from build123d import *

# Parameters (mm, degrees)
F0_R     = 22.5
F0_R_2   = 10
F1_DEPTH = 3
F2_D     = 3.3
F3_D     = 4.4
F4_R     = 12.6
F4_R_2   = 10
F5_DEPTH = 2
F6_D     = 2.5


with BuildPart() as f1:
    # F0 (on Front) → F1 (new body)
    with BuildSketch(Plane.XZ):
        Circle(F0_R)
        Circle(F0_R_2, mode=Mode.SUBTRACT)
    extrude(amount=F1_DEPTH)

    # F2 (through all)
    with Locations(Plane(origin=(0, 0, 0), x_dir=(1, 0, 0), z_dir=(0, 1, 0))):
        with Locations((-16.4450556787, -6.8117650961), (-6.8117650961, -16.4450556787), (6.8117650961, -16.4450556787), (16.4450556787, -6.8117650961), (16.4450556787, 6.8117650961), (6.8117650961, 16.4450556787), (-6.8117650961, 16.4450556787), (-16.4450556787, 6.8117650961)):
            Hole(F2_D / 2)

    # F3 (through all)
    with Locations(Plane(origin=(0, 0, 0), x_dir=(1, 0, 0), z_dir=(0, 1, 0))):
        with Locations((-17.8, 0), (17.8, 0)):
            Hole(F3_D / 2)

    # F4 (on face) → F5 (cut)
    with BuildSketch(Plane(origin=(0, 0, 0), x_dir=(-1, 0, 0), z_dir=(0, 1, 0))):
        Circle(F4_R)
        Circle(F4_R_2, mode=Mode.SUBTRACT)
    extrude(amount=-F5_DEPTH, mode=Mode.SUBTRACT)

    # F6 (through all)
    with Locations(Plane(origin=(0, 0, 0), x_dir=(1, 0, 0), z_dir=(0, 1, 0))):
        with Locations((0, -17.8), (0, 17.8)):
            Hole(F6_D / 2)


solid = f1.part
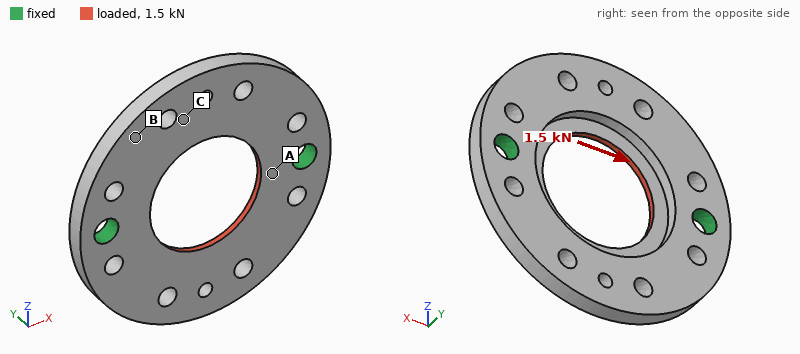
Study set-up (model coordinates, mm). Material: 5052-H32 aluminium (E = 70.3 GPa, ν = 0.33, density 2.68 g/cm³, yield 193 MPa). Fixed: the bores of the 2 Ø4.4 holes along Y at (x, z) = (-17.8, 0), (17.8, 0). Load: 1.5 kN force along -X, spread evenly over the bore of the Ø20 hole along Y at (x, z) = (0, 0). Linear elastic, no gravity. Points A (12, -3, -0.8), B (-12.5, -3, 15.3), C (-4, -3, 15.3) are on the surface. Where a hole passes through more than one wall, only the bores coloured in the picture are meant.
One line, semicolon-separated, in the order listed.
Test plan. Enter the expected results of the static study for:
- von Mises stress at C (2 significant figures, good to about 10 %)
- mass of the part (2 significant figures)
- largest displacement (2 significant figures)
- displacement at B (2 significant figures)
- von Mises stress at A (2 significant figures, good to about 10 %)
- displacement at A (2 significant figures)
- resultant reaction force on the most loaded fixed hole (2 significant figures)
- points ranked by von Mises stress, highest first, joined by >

12 MPa; 8.4 g; 10 µm; 7.9 µm; 40 MPa; 2.8 µm; 750 N; A > C > B
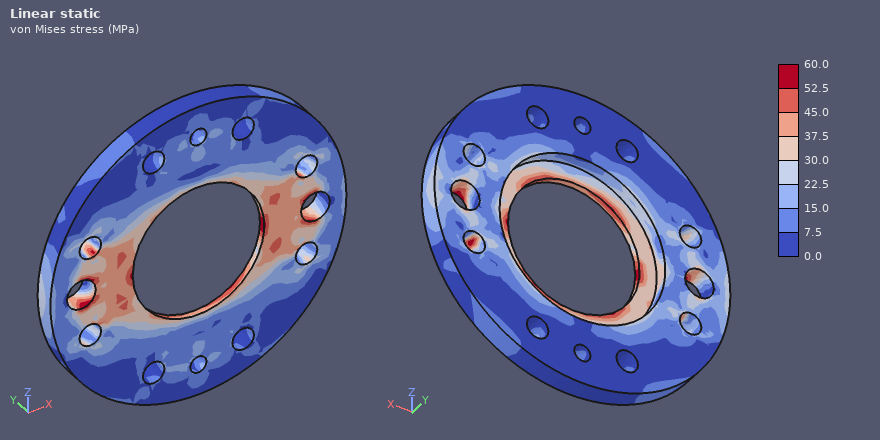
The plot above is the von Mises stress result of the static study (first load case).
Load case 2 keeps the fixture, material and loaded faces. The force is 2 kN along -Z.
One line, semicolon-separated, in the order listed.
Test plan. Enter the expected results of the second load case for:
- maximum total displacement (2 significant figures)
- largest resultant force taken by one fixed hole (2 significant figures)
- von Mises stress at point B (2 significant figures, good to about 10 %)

55 µm; 1.0 kN; 20 MPa
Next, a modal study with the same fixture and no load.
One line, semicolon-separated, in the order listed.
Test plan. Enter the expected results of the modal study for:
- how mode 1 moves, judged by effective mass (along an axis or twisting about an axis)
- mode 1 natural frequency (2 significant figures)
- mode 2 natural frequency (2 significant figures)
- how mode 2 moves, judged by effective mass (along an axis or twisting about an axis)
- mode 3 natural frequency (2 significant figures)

twisting about X; 4400 Hz; 4600 Hz; along Y; 12 kHz
